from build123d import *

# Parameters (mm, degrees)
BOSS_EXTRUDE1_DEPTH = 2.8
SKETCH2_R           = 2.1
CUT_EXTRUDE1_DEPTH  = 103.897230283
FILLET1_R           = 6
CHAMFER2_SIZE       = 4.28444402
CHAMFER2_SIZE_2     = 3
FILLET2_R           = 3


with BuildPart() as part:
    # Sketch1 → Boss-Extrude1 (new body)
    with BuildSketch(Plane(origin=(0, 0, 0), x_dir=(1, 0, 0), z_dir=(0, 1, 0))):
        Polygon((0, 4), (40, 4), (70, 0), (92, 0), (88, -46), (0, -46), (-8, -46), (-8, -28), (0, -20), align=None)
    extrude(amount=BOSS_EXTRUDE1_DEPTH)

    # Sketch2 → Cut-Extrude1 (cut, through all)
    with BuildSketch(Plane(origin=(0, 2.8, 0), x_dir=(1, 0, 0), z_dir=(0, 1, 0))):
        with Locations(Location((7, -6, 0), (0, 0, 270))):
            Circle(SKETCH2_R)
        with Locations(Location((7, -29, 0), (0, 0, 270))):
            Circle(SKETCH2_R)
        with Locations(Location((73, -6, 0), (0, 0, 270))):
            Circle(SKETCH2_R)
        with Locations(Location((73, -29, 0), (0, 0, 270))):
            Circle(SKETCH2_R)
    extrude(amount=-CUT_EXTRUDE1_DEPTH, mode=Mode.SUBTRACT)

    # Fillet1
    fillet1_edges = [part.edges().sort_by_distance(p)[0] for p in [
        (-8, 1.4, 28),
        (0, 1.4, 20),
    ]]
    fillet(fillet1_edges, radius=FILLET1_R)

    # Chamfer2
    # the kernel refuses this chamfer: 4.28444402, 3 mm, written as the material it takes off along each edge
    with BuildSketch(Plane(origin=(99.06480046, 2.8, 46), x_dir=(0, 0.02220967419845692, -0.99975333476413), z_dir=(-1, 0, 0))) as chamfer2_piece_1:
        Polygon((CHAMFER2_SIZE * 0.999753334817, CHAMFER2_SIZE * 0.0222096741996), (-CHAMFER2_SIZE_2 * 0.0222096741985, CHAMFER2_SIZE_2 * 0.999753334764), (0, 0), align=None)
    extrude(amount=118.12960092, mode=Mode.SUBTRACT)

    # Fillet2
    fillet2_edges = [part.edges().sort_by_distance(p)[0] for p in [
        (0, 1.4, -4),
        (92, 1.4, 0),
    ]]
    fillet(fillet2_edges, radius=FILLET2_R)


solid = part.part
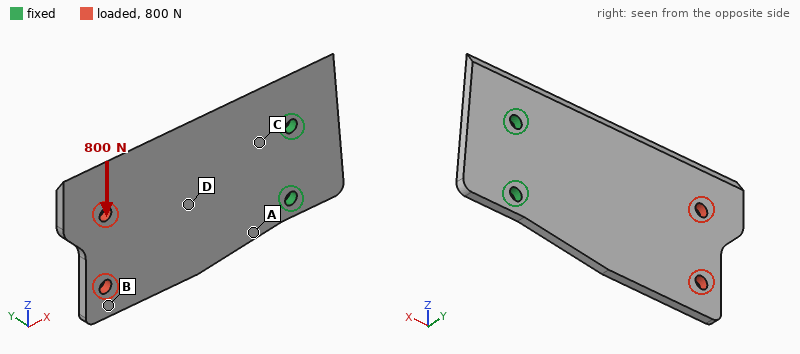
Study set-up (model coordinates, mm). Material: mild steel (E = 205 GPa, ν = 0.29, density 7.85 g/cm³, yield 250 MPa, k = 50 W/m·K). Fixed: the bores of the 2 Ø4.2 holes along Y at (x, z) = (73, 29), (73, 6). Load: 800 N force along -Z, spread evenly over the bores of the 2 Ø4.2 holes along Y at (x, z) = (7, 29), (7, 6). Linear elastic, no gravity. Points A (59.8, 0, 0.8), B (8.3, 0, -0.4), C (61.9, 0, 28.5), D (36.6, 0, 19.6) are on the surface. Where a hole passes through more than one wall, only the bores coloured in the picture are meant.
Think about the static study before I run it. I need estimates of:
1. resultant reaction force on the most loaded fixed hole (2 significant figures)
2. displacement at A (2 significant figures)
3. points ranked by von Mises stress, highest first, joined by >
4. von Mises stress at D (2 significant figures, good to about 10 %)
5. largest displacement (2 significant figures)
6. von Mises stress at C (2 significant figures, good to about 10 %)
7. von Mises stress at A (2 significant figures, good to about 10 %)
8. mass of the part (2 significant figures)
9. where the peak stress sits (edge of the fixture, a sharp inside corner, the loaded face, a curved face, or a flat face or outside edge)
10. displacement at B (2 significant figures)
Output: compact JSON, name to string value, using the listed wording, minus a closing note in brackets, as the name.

{"resultant reaction force on the most loaded fixed hole": "2.2 kN", "displacement at A": "6.4 µm", "points ranked by von Mises stress, highest first, joined by >": "A > C > D > B", "von Mises stress at D": "17 MPa", "largest displacement": "43 µm", "von Mises stress at C": "31 MPa", "von Mises stress at A": "45 MPa", "mass of the part": "94 g", "where the peak stress sits": "edge of the fixture", "displacement at B": "33 µm"}
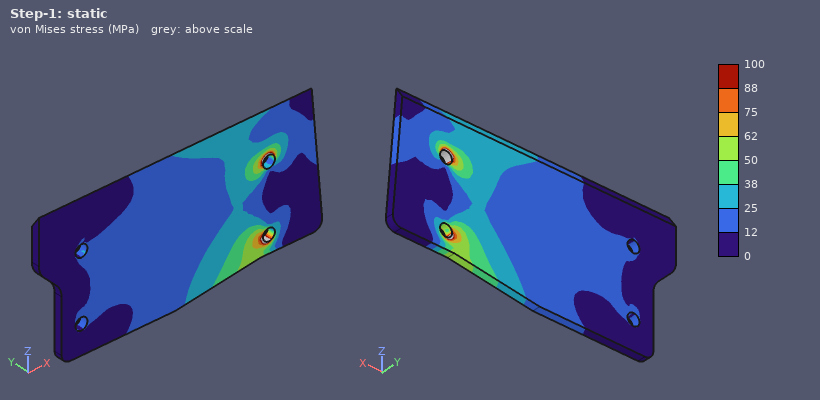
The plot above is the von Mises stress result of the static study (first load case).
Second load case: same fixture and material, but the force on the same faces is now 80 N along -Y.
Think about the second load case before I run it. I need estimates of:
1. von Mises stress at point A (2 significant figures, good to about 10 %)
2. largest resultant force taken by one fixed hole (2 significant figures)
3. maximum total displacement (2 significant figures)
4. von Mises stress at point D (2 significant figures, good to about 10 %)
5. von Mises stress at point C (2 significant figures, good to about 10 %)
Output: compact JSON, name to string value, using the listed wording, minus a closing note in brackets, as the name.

{"von Mises stress at point A": "78 MPa", "largest resultant force taken by one fixed hole": "41 N", "maximum total displacement": "0.58 mm", "von Mises stress at point D": "36 MPa", "von Mises stress at point C": "65 MPa"}
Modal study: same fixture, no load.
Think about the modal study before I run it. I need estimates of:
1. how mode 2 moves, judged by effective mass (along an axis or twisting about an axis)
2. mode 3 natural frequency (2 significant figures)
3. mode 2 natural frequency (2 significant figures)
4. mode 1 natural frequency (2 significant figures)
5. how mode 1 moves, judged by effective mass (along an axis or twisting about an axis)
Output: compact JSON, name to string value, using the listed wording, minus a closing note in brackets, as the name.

{"how mode 2 moves, judged by effective mass": "twisting about X", "mode 3 natural frequency": "2400 Hz", "mode 2 natural frequency": "1400 Hz", "mode 1 natural frequency": "390 Hz", "how mode 1 moves, judged by effective mass": "along Y"}
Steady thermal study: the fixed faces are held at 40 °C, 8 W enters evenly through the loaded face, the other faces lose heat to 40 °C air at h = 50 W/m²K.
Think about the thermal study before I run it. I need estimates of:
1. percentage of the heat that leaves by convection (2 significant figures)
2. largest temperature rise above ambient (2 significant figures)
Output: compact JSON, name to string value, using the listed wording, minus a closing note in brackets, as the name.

{"percentage of the heat that leaves by convection": "78 %", "largest temperature rise above ambient": "39 K"}
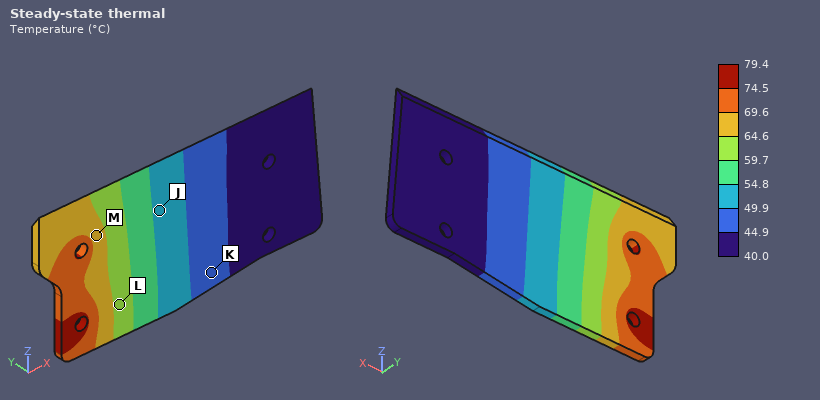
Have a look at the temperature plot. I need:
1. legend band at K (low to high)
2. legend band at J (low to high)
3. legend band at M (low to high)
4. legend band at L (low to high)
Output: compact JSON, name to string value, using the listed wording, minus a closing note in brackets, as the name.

{"legend band at K": "44.9 to 49.9 °C", "legend band at J": "49.9 to 54.8 °C", "legend band at M": "64.6 to 69.6 °C", "legend band at L": "59.7 to 64.6 °C"}
